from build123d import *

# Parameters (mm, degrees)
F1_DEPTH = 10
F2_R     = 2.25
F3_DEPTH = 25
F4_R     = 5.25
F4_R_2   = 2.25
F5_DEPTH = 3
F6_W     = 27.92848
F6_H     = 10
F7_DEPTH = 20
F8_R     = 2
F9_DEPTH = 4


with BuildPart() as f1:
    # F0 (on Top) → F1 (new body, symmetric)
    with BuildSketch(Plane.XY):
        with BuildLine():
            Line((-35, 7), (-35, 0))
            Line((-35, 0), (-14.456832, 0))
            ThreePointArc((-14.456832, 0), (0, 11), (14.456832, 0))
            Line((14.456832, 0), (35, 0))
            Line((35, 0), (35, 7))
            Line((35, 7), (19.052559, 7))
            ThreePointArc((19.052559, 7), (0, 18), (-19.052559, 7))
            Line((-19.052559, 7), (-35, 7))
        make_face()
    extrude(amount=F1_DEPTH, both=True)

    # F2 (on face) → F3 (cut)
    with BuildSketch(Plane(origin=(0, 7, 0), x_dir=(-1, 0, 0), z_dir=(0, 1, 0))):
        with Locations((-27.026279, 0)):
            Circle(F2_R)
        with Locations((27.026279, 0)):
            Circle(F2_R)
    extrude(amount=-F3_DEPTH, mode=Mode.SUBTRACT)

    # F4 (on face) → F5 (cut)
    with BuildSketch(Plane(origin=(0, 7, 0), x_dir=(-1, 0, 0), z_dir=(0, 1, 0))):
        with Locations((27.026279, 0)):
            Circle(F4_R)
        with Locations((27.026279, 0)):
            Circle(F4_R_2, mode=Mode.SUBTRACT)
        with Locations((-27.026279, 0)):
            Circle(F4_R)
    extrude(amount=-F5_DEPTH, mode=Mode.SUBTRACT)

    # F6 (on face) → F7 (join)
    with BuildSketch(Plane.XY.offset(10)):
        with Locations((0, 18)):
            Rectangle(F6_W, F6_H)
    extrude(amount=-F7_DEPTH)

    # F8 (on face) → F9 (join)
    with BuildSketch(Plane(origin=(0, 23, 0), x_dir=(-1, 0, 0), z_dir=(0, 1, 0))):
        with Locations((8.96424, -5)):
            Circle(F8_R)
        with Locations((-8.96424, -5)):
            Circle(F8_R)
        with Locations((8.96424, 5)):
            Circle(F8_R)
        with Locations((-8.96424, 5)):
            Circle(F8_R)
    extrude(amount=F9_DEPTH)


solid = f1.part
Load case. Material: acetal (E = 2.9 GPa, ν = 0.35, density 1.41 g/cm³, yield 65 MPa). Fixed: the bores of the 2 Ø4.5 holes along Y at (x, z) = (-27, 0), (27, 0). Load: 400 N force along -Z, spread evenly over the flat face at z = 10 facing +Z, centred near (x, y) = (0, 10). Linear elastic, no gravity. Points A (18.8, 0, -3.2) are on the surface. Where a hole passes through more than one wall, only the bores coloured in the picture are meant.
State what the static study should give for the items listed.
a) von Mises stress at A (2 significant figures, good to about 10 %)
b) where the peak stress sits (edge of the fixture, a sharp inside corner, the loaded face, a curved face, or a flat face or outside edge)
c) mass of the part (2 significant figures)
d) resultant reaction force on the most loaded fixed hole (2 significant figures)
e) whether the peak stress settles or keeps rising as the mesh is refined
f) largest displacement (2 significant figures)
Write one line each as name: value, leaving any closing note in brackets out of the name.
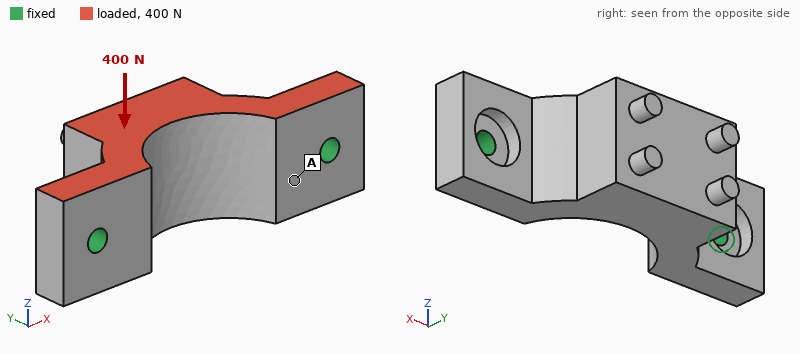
von Mises stress at A: 5.3 MPa
where the peak stress sits: edge of the fixture
mass of the part: 20 g
resultant reaction force on the most loaded fixed hole: 200 N
whether the peak stress settles or keeps rising as the mesh is refined: keeps rising
largest displacement: 0.52 mm
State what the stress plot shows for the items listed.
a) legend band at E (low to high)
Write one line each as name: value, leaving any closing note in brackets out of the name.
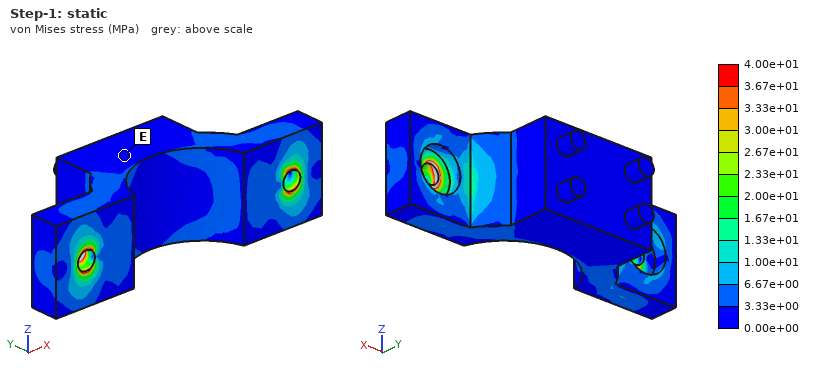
legend band at E: 0.00e+00 to 3.33e+00 MPa
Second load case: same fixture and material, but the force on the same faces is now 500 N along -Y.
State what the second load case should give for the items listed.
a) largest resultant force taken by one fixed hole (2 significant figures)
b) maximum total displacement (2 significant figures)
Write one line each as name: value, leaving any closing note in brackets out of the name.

largest resultant force taken by one fixed hole: 310 N
maximum total displacement: 0.61 mm
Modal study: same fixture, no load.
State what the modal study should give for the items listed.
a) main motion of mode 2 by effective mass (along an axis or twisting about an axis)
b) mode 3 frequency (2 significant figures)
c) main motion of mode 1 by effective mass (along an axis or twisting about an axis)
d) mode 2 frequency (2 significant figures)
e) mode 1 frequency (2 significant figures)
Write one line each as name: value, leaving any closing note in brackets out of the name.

main motion of mode 2 by effective mass: along Y
mode 3 frequency: 4300 Hz
main motion of mode 1 by effective mass: along Z
mode 2 frequency: 3200 Hz
mode 1 frequency: 1200 Hz
